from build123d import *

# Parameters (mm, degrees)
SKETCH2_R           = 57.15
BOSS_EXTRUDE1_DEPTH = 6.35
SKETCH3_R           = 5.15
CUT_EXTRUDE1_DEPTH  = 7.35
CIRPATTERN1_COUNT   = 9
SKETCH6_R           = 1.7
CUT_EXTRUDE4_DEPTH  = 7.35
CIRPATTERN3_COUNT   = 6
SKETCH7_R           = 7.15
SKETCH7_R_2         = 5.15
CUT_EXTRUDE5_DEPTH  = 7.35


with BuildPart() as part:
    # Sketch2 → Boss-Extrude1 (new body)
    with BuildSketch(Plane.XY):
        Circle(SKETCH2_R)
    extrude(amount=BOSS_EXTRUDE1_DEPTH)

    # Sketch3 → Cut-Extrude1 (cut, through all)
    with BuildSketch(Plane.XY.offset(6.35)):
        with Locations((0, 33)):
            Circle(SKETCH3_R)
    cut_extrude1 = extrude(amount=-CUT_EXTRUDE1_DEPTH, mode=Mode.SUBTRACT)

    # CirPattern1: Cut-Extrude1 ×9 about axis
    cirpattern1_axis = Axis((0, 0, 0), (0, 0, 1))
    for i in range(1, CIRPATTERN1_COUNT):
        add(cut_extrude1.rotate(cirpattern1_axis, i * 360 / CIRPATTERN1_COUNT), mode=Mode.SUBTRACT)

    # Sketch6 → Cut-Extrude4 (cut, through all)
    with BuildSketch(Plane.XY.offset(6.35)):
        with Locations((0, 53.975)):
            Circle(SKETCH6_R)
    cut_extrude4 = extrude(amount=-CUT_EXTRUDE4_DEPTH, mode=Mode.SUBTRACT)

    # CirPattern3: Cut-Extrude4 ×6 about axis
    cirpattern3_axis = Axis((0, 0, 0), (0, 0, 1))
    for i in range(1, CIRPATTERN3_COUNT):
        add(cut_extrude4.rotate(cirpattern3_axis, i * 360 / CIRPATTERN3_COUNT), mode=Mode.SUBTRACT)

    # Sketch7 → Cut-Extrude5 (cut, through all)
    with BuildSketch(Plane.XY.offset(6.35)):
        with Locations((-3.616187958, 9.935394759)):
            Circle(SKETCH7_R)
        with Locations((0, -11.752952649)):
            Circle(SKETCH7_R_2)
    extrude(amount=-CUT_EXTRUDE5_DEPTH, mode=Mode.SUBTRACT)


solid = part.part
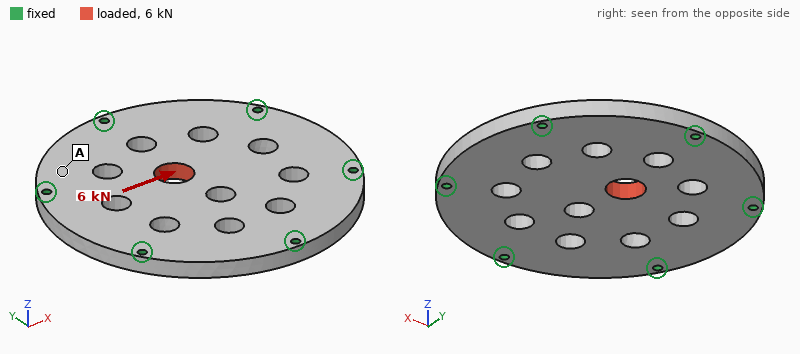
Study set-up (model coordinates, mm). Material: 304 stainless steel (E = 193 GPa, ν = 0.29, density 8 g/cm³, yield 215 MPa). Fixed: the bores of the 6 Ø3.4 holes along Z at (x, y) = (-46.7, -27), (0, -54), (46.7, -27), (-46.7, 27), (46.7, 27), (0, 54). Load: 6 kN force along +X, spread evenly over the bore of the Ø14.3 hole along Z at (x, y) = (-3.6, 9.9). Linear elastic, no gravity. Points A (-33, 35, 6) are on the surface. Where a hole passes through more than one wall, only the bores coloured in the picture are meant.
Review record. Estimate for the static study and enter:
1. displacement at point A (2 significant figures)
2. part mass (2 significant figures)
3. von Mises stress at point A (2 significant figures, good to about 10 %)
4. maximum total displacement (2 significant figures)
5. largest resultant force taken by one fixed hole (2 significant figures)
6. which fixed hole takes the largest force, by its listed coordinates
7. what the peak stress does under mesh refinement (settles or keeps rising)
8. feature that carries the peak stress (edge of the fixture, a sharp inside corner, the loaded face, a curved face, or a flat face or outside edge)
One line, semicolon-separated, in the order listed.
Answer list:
1.2 µm; 470 g; 5.8 MPa; 4.3 µm; 1.6 kN; (-46.7, 27); keeps rising; edge of the fixture
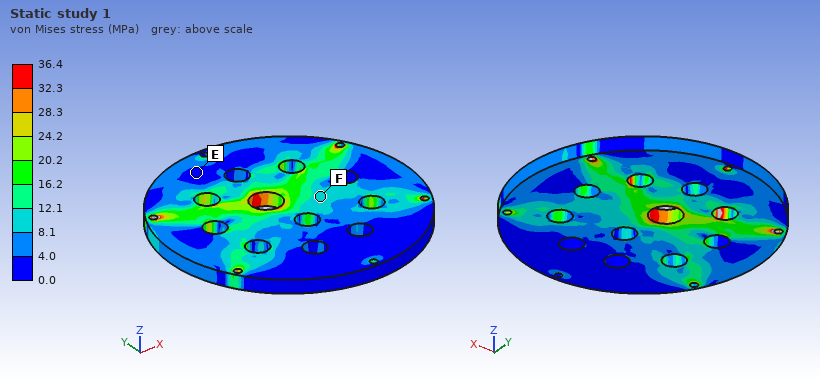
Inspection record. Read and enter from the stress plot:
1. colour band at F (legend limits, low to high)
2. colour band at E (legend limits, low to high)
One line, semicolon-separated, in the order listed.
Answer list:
8.1 to 12.1 MPa; 0.0 to 4.0 MPa
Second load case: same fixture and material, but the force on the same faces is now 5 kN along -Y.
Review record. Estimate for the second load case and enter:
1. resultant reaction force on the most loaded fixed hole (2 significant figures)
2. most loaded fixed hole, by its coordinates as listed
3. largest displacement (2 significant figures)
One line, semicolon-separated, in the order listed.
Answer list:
1.5 kN; (0, 54); 3.9 µm
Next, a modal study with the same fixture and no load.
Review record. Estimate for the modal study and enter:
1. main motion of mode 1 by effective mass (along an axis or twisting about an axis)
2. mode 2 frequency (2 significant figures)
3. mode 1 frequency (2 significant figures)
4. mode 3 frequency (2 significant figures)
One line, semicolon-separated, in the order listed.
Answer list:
along Z; 7400 Hz; 3700 Hz; 7400 Hz
